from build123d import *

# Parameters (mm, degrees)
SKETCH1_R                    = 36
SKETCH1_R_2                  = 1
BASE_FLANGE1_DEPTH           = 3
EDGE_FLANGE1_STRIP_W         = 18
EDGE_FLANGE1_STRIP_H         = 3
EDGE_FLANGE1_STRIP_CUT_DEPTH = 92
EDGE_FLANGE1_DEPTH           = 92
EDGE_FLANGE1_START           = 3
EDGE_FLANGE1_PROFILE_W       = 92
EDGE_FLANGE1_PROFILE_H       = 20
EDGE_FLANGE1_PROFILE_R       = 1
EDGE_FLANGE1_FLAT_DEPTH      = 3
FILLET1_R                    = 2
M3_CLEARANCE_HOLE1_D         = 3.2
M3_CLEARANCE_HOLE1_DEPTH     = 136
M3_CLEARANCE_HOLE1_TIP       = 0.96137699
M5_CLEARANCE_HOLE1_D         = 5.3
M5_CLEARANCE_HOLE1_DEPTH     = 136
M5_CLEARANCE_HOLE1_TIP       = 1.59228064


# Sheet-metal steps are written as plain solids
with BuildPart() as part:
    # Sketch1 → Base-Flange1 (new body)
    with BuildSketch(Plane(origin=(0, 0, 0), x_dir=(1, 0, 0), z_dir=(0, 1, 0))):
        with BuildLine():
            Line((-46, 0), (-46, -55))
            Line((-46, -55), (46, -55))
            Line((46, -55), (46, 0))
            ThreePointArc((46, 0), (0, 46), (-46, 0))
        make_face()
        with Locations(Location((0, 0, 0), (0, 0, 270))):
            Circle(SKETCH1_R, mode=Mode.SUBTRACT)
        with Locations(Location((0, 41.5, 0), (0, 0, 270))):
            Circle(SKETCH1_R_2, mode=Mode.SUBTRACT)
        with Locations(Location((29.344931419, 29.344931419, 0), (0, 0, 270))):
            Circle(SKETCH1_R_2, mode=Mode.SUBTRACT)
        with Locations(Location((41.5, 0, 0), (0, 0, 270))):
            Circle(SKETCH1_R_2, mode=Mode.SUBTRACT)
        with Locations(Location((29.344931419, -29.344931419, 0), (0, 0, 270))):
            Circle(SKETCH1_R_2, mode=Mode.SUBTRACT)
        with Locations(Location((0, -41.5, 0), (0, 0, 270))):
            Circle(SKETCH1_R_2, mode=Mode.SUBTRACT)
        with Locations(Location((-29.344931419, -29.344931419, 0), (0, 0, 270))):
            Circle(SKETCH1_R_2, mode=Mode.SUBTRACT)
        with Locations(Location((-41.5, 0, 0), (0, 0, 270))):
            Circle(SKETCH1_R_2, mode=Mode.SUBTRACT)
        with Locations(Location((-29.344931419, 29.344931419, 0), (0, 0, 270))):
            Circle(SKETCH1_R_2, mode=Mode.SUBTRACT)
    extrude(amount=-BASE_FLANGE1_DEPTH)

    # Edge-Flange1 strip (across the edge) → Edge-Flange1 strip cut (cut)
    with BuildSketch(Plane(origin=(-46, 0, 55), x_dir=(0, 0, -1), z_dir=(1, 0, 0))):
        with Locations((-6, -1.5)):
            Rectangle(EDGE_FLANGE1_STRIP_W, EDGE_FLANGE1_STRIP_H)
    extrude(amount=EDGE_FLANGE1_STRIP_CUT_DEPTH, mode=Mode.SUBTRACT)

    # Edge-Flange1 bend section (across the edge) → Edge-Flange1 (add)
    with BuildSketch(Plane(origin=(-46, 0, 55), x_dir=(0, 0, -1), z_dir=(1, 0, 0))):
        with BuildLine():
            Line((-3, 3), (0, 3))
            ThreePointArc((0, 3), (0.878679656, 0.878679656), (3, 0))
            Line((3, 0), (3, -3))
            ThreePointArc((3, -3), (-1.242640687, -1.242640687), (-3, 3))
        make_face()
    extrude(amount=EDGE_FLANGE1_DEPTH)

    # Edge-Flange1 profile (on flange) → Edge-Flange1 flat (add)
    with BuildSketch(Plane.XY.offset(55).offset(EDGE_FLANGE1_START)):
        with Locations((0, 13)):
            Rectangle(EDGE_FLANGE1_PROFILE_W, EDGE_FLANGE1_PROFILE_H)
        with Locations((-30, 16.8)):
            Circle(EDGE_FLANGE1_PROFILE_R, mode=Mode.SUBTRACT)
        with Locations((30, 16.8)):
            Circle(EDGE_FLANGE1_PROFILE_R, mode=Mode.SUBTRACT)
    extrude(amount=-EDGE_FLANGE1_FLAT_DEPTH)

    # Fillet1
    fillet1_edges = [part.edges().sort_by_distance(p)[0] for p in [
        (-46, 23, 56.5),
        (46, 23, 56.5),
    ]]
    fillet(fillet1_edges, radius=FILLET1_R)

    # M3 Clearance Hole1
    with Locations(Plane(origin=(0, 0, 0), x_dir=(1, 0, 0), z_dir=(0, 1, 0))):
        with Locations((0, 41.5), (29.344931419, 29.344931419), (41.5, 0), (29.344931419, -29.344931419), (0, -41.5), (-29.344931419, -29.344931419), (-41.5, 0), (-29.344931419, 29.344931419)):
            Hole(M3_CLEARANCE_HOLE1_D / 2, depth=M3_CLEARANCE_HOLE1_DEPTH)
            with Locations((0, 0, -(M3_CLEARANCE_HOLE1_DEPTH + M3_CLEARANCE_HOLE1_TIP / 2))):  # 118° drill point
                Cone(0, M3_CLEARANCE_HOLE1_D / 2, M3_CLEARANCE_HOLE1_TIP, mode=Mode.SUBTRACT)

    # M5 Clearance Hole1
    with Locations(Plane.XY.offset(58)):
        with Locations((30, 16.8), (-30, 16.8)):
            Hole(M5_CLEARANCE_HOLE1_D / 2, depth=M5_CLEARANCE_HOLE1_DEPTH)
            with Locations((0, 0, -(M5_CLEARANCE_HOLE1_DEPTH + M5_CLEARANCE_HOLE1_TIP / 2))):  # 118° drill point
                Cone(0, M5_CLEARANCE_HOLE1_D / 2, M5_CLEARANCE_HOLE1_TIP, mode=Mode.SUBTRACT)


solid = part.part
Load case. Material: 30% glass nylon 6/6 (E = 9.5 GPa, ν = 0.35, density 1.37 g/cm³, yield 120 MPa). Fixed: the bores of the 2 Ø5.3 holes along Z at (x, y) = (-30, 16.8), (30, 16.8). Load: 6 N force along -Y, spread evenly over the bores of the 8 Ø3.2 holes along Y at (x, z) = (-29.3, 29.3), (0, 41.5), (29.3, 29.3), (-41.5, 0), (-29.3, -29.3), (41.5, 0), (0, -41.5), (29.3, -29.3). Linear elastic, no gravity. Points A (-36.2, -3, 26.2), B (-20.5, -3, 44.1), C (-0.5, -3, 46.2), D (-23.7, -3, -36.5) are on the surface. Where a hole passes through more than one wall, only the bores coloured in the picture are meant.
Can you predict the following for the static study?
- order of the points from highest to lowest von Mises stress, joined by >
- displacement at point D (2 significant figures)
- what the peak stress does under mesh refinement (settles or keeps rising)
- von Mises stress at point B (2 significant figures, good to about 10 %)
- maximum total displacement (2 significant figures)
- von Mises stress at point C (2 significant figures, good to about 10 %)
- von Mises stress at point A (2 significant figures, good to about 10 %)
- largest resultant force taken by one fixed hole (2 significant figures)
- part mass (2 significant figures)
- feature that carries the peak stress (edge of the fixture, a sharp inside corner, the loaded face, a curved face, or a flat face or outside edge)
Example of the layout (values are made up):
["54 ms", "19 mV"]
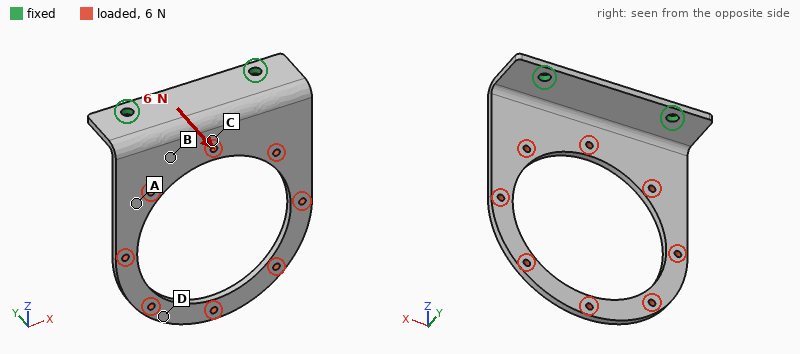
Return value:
["A > B > C > D", "1.1 mm", "keeps rising", "1.9 MPa", "1.3 mm", "1.0 MPa", "3.1 MPa", "3.2 N", "26 g", "edge of the fixture"]
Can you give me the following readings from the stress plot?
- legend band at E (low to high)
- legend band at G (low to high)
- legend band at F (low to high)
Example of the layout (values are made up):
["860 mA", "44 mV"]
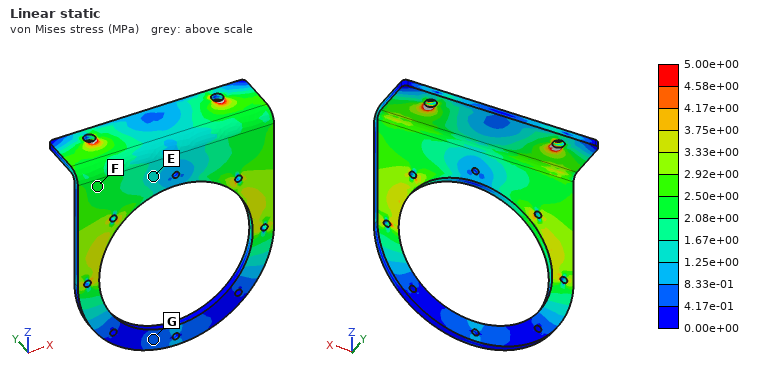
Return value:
["1.25e+00 to 1.67e+00 MPa", "4.17e-01 to 8.33e-01 MPa", "2.08e+00 to 2.50e+00 MPa"]
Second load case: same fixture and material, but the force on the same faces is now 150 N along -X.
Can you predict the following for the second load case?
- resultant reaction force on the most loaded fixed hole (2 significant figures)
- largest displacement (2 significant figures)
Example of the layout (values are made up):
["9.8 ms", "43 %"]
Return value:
["160 N", "1.2 mm"]
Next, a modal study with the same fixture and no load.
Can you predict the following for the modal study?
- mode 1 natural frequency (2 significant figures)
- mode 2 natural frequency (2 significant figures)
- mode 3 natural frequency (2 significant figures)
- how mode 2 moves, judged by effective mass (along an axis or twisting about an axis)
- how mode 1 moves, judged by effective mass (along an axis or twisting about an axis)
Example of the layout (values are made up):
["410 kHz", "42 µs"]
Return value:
["130 Hz", "320 Hz", "560 Hz", "twisting about Z", "along Y"]
